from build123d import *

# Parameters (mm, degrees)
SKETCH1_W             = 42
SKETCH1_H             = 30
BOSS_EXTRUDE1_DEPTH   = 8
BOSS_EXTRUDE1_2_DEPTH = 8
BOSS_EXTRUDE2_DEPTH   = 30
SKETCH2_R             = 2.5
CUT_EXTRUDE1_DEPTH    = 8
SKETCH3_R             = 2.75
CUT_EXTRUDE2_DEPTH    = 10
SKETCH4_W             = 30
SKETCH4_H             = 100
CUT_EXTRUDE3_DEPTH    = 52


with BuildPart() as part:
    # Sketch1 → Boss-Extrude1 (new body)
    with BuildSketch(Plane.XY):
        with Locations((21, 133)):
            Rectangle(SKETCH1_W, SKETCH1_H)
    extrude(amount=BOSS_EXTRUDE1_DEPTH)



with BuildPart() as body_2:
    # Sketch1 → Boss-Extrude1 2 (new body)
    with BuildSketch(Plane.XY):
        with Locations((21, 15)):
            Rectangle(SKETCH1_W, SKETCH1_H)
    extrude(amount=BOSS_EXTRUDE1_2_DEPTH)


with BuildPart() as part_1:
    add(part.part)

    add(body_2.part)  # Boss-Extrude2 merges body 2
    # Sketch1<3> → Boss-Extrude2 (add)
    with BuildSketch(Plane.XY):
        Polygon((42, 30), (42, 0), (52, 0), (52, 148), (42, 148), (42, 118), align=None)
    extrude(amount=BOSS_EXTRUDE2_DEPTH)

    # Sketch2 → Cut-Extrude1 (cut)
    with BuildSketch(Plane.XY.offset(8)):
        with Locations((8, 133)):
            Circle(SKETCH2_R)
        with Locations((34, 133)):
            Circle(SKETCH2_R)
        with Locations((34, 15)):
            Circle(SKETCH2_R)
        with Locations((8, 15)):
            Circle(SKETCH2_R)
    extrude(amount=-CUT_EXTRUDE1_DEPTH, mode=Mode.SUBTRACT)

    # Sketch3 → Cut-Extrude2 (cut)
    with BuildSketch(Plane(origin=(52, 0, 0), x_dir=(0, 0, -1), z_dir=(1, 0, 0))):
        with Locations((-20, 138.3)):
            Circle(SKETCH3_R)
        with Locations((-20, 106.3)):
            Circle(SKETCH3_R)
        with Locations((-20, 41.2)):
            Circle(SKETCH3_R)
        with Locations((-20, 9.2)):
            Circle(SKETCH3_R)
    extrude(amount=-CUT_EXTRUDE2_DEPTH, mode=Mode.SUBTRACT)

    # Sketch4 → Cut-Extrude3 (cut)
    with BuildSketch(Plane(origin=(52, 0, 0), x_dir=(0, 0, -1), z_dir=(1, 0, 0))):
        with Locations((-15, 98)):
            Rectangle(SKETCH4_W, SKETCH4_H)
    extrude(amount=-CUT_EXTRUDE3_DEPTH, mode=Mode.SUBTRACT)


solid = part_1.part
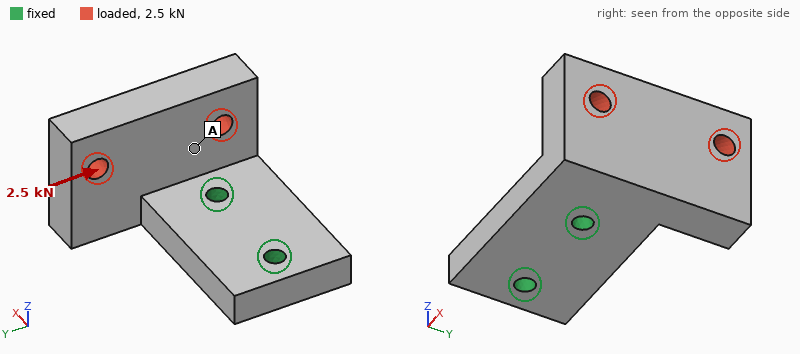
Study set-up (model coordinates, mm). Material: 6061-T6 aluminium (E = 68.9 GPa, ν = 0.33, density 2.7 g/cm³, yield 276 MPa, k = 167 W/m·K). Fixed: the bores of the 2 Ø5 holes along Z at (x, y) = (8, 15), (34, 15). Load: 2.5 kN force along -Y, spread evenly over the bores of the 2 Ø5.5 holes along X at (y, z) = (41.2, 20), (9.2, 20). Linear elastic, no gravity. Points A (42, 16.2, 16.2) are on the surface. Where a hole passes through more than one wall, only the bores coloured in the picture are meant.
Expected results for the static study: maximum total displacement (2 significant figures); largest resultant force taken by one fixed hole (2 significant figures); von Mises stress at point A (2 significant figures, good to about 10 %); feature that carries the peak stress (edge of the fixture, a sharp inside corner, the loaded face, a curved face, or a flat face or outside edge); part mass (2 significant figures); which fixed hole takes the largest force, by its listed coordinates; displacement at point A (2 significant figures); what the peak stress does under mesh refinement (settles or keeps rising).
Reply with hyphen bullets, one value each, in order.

- 0.17 mm
- 3.4 kN
- 26 MPa
- edge of the fixture
- 64 g
- (34, 15)
- 0.056 mm
- keeps rising
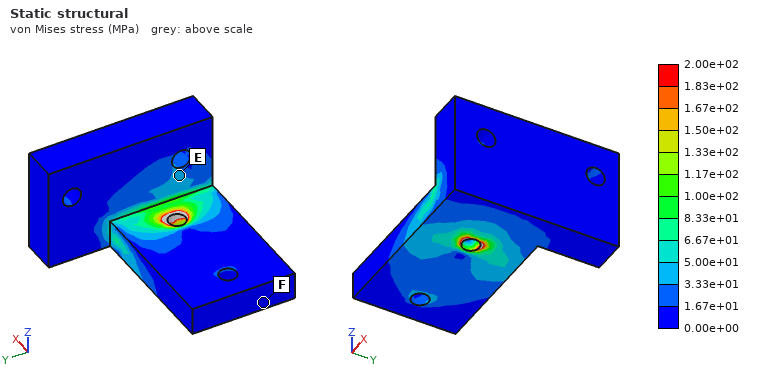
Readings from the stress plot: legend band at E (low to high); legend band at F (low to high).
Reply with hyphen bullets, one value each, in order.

- 3.33e+01 to 5.00e+01 MPa
- 0.00e+00 to 1.67e+01 MPa
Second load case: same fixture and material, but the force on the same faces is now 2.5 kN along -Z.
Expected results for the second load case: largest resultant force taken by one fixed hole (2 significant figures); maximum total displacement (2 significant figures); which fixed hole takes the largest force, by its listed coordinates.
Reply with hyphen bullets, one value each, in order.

- 2.9 kN
- 0.17 mm
- (34, 15)
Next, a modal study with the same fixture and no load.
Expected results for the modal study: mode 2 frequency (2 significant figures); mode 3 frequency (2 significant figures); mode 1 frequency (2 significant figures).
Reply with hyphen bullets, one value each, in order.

- 4400 Hz
- 7400 Hz
- 3500 Hz
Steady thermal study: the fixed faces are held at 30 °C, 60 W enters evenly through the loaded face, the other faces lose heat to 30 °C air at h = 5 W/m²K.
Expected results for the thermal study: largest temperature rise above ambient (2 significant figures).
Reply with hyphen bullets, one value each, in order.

- 42 K
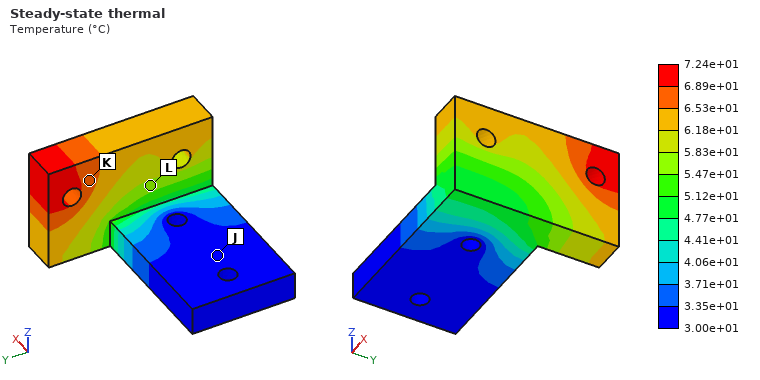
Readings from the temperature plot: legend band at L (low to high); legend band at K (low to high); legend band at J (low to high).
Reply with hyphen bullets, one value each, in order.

- 5.47e+01 to 5.83e+01 °C
- 6.53e+01 to 6.89e+01 °C
- 3.00e+01 to 3.35e+01 °C
